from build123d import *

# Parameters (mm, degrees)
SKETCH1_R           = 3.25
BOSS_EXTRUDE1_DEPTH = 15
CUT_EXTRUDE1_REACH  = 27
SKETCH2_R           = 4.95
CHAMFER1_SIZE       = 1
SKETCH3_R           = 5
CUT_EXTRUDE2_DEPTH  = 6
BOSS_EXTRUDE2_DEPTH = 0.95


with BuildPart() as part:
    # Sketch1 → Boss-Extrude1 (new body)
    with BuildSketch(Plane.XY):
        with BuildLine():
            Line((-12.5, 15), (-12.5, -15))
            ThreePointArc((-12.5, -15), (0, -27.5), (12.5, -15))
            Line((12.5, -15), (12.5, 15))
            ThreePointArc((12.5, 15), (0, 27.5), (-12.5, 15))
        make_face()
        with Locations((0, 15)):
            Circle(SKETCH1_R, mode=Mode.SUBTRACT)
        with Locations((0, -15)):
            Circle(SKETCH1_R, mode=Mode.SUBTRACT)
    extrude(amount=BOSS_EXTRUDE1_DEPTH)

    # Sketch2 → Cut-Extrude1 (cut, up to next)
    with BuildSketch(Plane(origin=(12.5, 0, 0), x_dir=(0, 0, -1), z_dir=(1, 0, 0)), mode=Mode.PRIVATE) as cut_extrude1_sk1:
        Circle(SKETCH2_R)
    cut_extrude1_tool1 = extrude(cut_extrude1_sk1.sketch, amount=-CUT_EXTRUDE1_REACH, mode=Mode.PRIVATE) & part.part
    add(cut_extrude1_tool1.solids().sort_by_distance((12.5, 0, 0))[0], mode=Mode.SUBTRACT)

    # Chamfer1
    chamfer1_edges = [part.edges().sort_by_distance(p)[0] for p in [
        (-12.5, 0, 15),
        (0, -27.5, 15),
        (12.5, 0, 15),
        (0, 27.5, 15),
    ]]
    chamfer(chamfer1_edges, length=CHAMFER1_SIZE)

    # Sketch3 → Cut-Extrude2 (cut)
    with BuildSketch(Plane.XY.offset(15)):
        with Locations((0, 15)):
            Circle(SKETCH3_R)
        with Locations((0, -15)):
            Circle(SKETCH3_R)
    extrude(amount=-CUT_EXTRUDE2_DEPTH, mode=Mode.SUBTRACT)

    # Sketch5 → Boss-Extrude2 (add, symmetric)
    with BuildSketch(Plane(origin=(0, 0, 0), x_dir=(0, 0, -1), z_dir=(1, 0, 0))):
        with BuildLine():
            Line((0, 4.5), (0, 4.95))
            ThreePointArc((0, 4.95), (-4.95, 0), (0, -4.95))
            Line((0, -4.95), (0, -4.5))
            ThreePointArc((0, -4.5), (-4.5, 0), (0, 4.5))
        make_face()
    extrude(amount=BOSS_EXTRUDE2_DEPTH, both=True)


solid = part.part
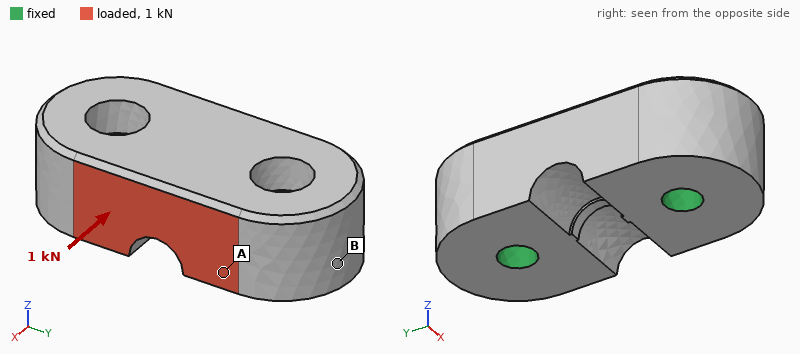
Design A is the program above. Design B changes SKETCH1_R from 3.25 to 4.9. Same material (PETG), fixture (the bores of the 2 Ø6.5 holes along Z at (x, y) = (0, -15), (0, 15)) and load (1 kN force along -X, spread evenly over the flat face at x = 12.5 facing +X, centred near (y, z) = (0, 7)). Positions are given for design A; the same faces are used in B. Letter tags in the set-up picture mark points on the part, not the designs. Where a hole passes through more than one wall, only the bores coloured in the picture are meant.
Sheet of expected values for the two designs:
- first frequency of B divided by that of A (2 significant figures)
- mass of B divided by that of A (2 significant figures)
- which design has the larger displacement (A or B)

1.4
0.95
A
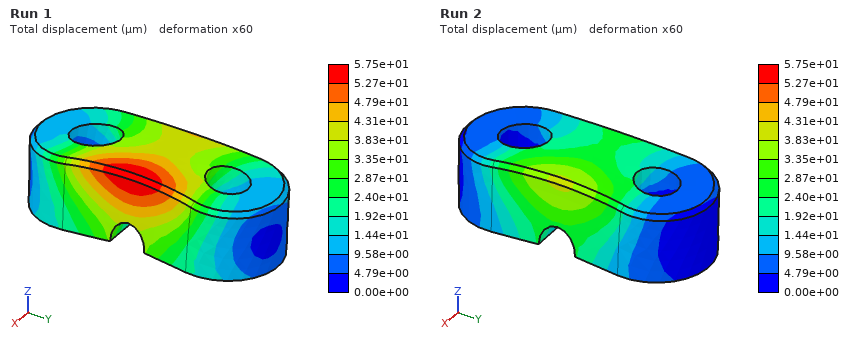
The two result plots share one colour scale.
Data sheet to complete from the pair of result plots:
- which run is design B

Run 2
